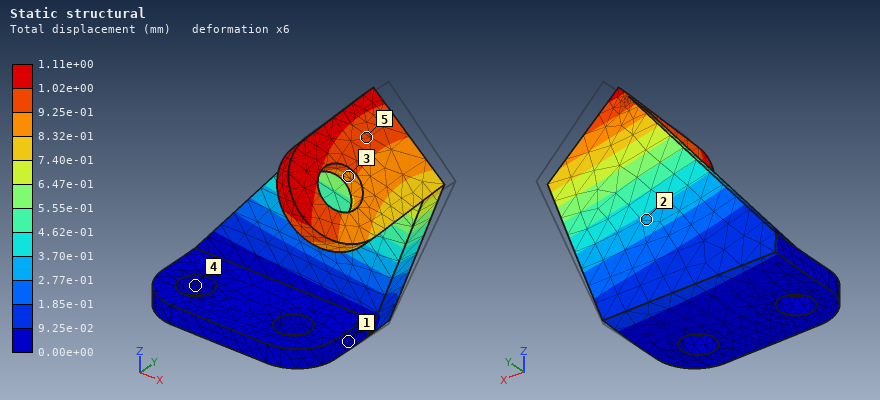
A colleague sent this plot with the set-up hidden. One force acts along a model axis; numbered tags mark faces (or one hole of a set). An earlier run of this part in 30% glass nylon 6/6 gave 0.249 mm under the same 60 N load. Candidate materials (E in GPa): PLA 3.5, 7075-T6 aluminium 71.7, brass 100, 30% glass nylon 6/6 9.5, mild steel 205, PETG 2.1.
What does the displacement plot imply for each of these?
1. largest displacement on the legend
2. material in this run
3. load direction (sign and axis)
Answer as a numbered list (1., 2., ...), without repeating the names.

1. 1.11e+00 mm
2. PETG
3. -Y
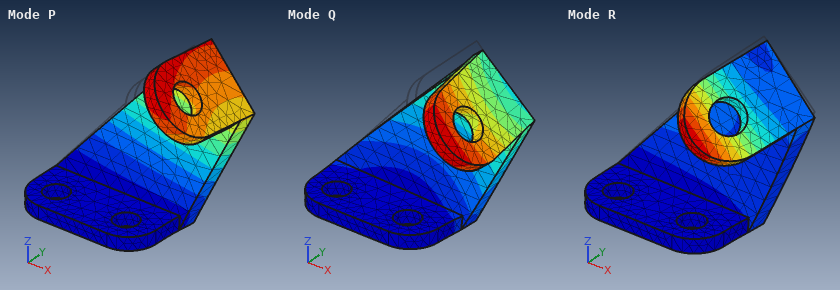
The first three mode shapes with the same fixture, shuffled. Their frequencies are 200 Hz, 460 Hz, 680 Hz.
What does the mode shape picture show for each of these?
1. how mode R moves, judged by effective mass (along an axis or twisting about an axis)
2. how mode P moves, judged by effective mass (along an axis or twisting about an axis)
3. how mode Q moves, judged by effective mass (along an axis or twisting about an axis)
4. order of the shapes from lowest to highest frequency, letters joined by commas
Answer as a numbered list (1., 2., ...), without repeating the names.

1. along Z
2. along Y
3. along X
4. P, Q, R
